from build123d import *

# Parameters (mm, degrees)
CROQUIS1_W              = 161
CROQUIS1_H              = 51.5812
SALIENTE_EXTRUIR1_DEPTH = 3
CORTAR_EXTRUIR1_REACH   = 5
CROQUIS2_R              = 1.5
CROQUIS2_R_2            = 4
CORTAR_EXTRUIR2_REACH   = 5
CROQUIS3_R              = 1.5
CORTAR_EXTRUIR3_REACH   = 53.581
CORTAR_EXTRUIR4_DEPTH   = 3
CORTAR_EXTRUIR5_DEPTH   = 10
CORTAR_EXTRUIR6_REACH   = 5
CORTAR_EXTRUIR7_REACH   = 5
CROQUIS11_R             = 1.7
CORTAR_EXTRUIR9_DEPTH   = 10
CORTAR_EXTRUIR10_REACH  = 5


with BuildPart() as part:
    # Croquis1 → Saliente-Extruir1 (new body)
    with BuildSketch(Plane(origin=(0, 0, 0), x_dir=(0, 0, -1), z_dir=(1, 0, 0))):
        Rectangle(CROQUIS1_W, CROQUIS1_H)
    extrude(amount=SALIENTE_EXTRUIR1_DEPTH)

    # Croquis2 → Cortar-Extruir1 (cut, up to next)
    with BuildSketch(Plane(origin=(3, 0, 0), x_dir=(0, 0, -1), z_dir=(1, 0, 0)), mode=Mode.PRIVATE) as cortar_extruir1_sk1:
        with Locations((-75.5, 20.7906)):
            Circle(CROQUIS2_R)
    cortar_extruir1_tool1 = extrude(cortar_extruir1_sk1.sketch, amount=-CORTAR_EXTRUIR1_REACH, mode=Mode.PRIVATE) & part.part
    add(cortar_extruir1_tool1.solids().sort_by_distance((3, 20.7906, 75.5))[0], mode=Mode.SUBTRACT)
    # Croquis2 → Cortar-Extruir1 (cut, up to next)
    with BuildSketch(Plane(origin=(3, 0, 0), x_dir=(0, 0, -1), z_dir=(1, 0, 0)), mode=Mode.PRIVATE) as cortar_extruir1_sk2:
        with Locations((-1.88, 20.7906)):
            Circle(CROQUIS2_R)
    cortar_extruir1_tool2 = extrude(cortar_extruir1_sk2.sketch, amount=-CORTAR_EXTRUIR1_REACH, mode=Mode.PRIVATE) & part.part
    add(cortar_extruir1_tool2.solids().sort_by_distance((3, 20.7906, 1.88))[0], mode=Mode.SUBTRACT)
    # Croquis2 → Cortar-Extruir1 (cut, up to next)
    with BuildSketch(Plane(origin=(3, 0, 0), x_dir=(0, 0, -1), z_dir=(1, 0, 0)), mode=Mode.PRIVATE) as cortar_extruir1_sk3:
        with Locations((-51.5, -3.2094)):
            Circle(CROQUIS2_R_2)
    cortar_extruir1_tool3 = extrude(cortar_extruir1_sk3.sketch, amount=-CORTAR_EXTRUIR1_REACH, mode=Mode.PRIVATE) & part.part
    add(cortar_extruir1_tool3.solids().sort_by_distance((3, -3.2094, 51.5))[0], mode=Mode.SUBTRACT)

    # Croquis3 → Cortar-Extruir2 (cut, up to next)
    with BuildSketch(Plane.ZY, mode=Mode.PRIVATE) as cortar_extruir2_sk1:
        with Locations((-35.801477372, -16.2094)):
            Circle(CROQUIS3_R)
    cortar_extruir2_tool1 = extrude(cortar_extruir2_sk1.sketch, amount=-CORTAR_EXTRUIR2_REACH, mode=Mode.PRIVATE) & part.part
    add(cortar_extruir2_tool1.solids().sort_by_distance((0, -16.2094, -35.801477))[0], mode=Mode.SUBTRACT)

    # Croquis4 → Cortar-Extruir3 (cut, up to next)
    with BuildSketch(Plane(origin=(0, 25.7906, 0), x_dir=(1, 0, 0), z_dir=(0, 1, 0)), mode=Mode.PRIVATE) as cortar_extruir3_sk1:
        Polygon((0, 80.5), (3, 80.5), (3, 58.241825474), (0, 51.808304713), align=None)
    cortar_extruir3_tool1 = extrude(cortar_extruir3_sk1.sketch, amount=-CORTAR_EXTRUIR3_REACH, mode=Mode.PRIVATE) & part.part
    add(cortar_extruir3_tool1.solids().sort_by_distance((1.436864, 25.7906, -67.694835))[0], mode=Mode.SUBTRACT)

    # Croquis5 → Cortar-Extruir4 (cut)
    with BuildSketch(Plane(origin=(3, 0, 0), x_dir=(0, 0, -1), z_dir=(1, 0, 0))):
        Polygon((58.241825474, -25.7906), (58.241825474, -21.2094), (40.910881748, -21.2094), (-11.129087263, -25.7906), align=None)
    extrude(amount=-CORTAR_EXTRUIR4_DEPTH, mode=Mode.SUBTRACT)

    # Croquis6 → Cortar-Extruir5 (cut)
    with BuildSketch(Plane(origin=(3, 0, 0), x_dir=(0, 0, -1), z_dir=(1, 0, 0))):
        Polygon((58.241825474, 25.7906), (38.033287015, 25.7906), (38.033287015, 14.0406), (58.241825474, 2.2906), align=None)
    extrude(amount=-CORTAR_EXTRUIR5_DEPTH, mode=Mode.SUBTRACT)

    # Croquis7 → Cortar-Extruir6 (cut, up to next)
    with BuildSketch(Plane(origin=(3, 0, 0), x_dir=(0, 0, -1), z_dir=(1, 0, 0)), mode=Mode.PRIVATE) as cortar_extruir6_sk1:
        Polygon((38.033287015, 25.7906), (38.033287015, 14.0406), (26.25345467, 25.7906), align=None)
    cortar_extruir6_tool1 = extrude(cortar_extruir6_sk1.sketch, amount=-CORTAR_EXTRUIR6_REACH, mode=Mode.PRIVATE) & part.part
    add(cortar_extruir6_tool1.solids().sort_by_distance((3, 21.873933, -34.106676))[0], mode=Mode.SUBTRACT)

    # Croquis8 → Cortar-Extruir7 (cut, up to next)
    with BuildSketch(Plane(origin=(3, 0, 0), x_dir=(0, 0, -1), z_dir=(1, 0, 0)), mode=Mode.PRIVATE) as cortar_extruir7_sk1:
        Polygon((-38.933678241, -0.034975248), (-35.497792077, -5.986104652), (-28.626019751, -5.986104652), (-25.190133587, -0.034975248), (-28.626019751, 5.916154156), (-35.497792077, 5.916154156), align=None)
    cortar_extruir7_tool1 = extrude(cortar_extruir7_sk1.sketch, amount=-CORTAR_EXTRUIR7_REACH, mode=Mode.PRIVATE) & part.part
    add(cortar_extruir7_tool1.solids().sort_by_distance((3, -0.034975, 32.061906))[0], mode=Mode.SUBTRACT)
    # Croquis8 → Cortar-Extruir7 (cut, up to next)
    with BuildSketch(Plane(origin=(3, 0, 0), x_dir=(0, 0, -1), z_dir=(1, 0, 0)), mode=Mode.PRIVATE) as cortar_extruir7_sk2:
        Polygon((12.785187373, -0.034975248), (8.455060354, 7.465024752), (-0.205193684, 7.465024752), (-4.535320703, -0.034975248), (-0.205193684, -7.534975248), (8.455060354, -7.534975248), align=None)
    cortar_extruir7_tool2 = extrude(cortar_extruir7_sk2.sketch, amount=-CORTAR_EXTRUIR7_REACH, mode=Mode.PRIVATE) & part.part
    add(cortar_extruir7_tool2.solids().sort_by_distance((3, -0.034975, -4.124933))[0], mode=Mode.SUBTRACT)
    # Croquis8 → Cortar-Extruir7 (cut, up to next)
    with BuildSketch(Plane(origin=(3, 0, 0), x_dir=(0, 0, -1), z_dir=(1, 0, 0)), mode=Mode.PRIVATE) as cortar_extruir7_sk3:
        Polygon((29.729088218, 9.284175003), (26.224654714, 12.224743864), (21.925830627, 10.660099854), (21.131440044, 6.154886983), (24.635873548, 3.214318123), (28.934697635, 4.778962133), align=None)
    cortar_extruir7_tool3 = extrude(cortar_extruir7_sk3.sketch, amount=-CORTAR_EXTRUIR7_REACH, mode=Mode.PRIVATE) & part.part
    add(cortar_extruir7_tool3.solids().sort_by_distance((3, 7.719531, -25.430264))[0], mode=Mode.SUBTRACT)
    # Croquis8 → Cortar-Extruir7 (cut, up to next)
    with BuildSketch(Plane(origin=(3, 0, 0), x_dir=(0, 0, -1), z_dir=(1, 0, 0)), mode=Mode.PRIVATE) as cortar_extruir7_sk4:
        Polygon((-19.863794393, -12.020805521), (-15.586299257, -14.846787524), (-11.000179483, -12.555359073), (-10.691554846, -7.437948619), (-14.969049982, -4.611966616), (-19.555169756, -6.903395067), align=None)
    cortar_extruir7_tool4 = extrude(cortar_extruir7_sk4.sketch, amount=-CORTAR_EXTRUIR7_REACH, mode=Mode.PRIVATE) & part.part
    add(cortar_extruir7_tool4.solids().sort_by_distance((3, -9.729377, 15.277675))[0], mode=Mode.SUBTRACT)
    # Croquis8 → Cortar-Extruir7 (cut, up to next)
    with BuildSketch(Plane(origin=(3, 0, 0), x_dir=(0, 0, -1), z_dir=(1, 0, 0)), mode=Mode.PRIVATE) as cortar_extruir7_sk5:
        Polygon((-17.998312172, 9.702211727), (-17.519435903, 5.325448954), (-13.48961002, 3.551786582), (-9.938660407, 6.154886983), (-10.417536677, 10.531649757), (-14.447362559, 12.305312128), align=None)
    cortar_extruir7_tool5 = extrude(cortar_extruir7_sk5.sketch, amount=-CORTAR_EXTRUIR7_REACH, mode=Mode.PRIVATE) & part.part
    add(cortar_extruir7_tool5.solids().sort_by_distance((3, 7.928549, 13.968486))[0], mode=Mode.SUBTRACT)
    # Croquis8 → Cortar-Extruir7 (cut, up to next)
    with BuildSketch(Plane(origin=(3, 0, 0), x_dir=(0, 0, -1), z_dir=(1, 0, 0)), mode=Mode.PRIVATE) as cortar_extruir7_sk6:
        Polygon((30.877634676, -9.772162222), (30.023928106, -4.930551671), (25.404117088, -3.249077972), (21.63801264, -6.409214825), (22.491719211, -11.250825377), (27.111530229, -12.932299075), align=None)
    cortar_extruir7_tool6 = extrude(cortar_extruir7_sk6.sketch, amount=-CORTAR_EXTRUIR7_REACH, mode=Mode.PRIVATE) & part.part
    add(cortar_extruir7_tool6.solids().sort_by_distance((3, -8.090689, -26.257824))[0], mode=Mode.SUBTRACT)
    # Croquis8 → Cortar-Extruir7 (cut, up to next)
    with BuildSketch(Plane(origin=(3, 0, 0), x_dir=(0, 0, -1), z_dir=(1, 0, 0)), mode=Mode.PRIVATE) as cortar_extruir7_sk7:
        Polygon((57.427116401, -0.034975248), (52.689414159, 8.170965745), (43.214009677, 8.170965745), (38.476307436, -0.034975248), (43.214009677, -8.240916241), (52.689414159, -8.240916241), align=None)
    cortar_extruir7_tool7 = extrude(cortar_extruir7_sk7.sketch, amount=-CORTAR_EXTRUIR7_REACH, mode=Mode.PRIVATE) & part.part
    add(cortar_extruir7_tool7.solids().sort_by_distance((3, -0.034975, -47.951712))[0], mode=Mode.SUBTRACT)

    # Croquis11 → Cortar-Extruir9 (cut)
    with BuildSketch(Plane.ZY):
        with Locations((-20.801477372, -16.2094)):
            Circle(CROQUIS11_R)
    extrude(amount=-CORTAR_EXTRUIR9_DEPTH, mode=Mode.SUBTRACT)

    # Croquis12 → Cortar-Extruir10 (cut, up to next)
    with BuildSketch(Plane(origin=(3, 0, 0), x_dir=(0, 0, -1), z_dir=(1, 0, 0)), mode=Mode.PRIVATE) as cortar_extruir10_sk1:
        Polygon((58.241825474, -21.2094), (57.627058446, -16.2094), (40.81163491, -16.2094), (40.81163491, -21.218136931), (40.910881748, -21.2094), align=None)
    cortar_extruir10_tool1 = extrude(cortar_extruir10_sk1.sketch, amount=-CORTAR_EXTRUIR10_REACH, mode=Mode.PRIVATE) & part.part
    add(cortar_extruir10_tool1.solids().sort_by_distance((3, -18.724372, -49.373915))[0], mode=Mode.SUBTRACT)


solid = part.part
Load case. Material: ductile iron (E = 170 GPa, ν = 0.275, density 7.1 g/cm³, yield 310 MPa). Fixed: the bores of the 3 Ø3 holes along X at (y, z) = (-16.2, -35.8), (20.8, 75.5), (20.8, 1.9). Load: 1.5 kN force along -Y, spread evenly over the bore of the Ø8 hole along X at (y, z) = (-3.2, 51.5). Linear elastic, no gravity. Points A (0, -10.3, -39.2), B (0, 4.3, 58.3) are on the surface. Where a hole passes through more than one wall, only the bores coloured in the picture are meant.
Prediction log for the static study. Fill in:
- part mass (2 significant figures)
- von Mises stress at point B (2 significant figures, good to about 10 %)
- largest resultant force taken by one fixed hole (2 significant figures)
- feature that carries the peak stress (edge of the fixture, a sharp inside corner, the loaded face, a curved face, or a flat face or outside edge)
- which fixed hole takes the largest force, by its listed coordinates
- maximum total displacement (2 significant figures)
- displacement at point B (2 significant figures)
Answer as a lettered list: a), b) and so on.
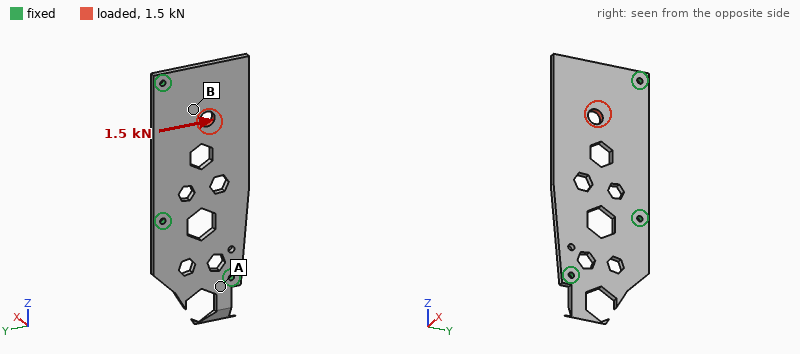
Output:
a) 120 g
b) 16 MPa
c) 1.1 kN
d) edge of the fixture
e) (20.8, 75.5)
f) 6.5 µm
g) 4.8 µm
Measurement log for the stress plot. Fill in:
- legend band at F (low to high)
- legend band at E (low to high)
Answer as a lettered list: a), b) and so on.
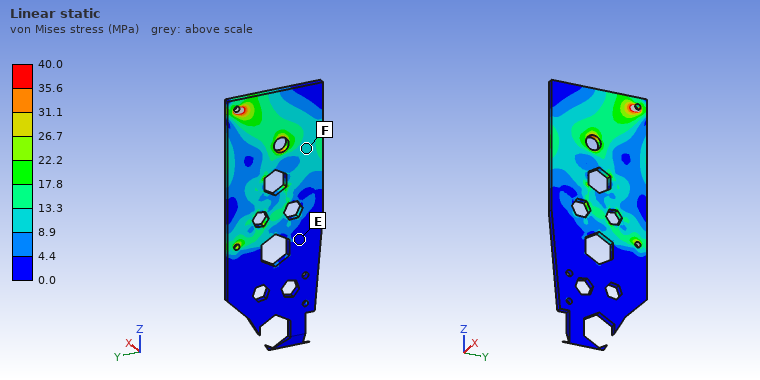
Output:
a) 8.9 to 13.3 MPa
b) 0.0 to 4.4 MPa
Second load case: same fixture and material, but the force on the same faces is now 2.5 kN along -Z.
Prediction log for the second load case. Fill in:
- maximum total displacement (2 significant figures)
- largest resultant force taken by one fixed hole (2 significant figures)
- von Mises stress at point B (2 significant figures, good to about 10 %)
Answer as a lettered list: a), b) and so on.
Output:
a) 8.8 µm
b) 1.1 kN
c) 24 MPa
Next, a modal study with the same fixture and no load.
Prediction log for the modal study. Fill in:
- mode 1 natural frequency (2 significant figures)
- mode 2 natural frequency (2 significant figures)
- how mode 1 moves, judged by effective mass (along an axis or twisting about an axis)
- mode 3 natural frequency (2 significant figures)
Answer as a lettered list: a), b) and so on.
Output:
a) 870 Hz
b) 2000 Hz
c) along X
d) 2800 Hz
